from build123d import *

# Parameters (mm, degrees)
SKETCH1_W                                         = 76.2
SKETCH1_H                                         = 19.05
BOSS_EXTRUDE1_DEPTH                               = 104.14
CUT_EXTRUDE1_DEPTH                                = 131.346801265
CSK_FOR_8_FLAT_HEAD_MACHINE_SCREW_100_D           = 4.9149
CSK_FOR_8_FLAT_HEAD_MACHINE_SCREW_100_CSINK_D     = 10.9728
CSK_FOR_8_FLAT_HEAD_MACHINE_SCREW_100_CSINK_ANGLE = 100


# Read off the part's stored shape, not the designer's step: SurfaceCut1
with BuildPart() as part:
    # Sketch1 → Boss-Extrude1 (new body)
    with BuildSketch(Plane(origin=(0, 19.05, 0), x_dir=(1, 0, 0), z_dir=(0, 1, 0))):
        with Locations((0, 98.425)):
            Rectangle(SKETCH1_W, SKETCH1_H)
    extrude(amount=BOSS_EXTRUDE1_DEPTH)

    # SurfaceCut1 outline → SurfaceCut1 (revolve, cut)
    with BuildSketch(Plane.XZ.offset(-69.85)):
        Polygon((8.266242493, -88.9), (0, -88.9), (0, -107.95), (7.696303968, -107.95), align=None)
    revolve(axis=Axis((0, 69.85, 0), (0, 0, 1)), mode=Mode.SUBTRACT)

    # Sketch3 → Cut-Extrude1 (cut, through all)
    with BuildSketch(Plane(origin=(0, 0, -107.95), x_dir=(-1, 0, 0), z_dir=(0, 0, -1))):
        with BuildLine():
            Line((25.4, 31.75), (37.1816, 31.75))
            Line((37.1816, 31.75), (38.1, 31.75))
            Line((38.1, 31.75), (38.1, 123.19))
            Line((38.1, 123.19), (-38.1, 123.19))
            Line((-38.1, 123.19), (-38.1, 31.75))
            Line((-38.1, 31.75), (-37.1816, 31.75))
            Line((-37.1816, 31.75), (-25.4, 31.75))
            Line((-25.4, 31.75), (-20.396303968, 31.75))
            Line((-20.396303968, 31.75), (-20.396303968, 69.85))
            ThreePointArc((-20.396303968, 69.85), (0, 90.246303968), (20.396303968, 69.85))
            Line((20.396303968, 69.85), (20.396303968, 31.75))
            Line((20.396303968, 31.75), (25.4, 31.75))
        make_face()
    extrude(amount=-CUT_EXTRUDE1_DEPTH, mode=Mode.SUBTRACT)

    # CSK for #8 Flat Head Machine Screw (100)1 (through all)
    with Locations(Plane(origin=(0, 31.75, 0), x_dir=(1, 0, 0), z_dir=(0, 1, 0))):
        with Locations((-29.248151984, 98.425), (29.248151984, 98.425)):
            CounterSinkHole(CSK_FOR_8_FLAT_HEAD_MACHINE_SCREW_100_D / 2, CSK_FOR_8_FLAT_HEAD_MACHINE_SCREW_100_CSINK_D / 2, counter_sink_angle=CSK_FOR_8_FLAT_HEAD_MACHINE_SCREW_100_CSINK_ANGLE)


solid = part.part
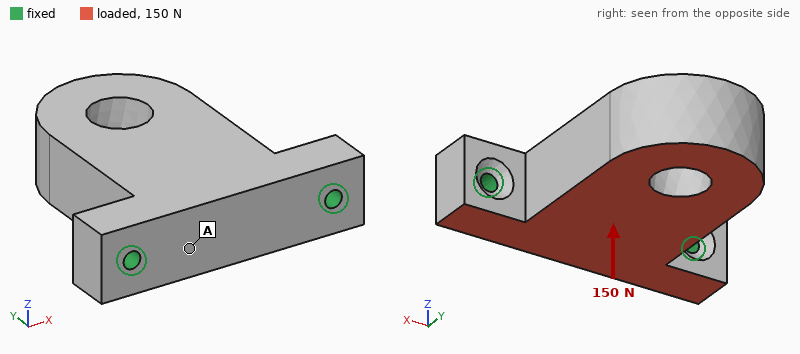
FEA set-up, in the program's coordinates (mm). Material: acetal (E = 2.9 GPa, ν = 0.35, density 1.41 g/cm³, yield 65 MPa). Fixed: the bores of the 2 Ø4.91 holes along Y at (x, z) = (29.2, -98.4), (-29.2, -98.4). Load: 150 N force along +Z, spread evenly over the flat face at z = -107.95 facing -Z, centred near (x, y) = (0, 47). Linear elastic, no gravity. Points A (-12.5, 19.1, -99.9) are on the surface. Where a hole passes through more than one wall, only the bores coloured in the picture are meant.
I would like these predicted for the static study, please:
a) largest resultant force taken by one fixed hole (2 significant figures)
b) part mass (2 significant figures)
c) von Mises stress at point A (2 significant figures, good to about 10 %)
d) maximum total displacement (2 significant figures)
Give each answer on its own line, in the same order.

75 N
79 g
1.1 MPa
0.26 mm
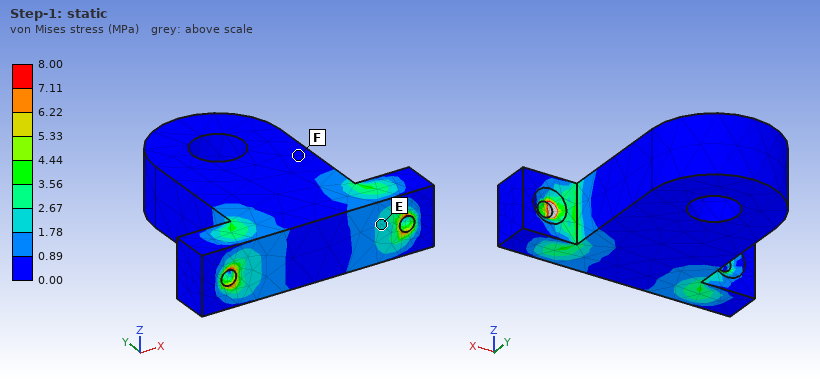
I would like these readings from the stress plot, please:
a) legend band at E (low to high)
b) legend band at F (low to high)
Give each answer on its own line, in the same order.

1.78 to 2.67 MPa
0.00 to 0.89 MPa
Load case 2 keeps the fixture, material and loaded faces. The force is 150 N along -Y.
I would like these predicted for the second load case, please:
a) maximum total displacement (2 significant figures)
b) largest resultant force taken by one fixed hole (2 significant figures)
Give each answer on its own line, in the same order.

99 µm
81 N
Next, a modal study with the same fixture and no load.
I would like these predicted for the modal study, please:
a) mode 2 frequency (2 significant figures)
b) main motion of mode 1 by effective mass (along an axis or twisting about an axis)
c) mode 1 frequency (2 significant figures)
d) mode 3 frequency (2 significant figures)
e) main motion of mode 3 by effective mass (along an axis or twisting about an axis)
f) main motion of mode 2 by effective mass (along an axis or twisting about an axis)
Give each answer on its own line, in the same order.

1600 Hz
along Z
540 Hz
2600 Hz
along Y
along X
